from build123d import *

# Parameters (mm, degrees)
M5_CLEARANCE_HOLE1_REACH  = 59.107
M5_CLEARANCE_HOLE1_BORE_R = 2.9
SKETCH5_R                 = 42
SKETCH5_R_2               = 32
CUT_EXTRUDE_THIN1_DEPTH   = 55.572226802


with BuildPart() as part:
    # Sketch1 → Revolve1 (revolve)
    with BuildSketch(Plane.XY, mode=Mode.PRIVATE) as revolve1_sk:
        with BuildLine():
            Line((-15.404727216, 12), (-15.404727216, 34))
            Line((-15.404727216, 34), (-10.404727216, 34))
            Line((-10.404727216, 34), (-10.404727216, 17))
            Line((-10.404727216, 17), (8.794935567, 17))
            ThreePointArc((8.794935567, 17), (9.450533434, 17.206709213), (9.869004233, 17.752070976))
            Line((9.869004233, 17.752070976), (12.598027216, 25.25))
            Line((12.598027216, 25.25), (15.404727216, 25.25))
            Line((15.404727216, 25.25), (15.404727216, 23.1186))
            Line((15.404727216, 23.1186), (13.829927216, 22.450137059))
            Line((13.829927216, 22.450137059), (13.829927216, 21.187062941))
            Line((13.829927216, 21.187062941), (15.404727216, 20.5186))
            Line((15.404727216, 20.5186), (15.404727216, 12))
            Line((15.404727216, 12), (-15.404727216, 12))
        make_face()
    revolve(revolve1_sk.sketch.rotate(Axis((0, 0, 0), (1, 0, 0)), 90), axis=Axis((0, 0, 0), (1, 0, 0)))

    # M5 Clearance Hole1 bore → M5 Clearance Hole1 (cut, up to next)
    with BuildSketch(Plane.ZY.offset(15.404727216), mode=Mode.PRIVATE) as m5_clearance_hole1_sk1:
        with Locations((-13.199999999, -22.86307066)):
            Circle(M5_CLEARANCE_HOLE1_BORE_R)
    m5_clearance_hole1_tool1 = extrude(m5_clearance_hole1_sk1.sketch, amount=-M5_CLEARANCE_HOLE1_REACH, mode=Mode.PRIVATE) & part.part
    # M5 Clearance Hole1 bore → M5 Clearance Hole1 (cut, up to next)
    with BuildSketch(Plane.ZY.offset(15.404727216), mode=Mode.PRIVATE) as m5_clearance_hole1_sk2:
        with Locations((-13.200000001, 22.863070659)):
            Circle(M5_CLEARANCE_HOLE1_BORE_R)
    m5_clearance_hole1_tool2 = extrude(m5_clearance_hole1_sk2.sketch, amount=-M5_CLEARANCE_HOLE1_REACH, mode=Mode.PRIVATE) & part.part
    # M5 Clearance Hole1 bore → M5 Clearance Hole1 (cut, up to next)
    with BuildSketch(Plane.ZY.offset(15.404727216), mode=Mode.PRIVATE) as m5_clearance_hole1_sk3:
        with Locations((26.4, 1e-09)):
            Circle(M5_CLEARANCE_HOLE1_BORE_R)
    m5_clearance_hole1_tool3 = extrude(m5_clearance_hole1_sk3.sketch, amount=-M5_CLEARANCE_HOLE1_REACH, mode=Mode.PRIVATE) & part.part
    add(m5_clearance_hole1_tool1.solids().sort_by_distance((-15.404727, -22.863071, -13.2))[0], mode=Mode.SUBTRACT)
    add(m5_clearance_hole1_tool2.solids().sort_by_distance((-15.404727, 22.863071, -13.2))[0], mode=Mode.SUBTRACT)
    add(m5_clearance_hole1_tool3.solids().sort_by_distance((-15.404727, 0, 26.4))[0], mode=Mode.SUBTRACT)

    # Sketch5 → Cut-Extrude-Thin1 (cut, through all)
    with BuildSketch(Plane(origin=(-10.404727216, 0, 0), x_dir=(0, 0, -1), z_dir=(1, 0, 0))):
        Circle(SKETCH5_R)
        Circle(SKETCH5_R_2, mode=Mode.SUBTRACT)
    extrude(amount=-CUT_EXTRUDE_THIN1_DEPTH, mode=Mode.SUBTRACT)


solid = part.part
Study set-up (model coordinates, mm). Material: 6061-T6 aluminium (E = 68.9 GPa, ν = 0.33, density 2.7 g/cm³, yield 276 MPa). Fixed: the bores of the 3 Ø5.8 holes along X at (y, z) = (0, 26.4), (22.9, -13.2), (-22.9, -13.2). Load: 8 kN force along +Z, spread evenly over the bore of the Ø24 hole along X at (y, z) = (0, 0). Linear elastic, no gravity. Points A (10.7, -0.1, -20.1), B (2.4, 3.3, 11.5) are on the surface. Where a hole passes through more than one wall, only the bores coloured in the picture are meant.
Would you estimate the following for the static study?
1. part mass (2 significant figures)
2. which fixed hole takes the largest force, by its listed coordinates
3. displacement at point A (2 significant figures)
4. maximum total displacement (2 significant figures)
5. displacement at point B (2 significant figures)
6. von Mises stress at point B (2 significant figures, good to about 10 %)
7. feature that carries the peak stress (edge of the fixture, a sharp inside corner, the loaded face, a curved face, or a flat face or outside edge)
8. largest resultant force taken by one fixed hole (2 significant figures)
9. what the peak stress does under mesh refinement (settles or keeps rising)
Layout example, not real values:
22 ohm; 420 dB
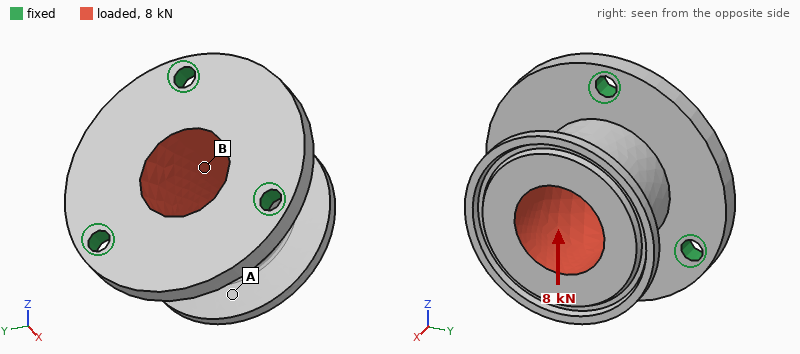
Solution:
79 g; (0, 26.4); 81 µm; 95 µm; 46 µm; 31 MPa; edge of the fixture; 4.0 kN; keeps rising
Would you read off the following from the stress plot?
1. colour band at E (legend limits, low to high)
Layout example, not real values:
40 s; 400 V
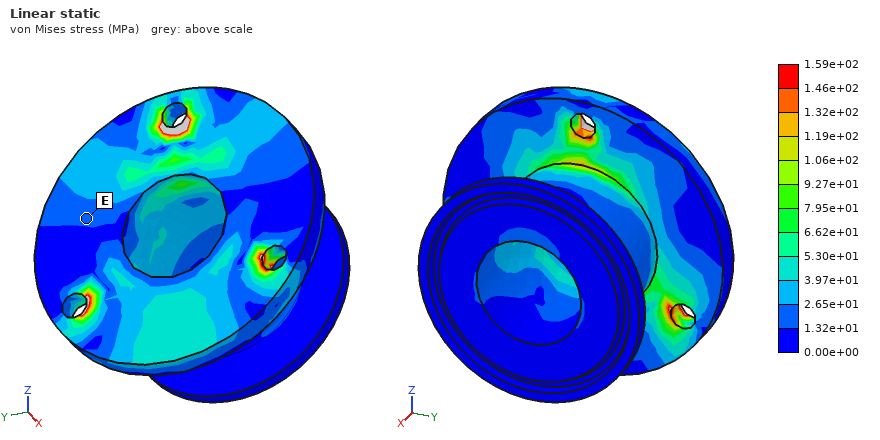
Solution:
1.32e+01 to 2.65e+01 MPa
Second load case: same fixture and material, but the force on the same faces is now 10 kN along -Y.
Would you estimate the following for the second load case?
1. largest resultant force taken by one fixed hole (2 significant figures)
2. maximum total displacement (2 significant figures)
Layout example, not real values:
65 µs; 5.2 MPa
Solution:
4.6 kN; 0.12 mm
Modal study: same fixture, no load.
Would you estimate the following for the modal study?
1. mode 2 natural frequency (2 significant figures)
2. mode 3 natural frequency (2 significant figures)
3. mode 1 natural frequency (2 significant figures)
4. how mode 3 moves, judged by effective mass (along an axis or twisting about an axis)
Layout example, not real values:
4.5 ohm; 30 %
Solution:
6200 Hz; 9000 Hz; 6200 Hz; along X
